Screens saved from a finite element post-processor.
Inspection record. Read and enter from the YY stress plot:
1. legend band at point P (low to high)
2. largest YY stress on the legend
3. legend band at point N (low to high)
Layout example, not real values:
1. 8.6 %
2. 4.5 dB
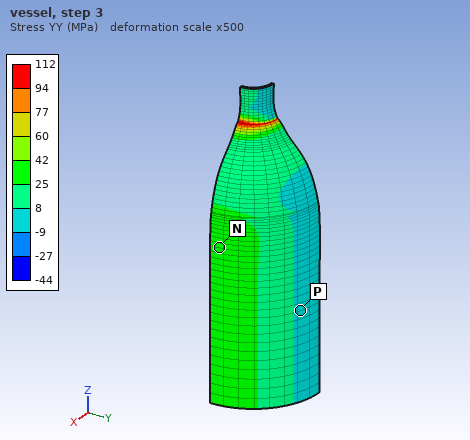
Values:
1. -9 to 8 MPa
2. 112 MPa
3. 25 to 42 MPa
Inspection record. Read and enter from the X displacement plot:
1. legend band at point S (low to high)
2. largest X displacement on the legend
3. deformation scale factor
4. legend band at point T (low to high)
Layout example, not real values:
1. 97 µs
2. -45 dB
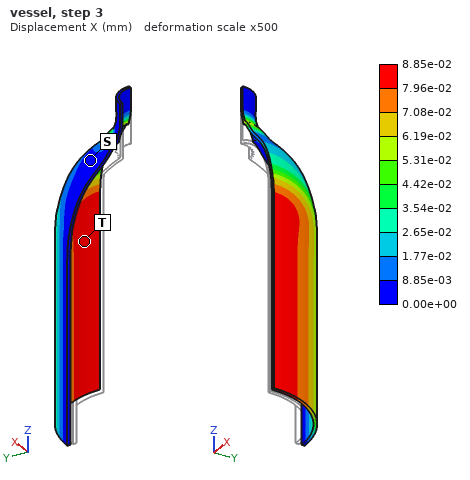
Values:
1. 0.00e+00 to 8.85e-03 mm
2. 8.85e-02 mm
3. 500
4. 7.96e-02 to 8.85e-02 mm
